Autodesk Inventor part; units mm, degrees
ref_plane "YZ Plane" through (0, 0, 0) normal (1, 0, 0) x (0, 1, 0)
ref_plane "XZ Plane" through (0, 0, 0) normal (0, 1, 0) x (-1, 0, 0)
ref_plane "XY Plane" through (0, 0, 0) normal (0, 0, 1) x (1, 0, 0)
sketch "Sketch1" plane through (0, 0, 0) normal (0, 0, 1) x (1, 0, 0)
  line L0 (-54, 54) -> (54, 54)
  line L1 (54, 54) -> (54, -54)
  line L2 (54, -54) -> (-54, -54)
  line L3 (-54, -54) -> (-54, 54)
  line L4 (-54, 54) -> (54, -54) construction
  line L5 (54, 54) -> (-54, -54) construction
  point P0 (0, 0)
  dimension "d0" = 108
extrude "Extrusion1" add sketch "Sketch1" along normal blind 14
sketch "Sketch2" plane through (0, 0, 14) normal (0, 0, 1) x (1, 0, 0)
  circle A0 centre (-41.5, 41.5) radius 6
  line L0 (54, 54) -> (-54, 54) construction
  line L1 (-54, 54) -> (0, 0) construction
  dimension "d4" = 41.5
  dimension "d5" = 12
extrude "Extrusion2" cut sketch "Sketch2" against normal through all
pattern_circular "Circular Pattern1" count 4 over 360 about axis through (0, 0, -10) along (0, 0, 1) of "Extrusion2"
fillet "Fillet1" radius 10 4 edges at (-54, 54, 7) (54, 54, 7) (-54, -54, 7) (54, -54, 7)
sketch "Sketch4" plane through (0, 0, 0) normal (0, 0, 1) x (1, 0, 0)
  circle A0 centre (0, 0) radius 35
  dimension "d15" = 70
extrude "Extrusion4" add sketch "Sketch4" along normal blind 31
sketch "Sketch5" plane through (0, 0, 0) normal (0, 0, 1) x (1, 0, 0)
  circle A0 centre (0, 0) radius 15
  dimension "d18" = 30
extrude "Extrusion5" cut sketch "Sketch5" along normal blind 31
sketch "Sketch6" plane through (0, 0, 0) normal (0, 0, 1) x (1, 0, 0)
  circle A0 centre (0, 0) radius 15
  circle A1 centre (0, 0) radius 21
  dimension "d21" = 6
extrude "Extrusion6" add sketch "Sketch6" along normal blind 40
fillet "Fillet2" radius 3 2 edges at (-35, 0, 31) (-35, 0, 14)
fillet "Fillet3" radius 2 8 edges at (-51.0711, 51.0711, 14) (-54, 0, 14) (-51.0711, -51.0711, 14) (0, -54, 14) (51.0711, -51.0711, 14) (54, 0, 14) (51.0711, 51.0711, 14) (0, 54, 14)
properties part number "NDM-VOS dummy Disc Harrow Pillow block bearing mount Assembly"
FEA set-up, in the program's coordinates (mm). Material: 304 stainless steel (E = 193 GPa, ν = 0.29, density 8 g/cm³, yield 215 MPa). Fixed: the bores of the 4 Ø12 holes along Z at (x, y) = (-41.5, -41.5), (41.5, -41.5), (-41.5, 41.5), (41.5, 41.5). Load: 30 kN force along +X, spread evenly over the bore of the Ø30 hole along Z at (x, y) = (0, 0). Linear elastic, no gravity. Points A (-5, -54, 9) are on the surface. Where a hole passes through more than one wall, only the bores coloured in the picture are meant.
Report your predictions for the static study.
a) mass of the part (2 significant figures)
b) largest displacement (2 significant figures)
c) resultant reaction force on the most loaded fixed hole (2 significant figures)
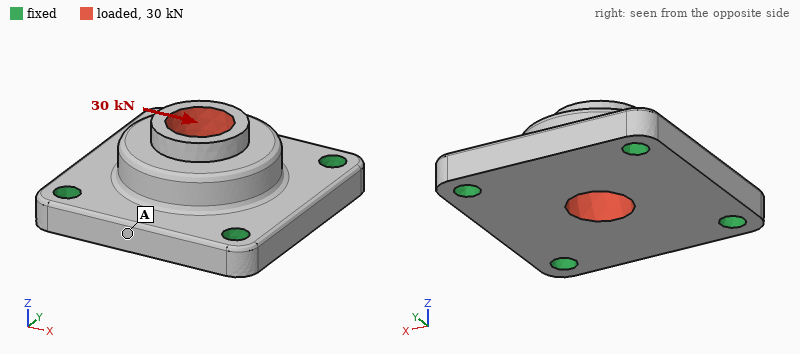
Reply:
1.6 kg
12 µm
8.6 kN
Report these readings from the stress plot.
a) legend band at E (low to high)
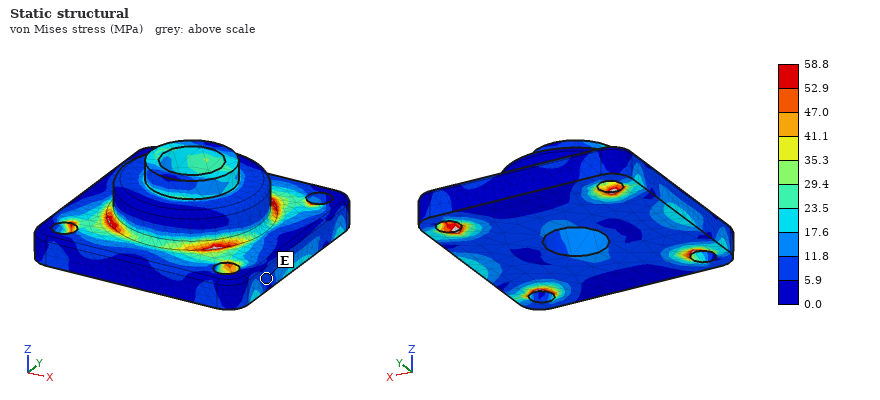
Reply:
5.9 to 11.8 MPa
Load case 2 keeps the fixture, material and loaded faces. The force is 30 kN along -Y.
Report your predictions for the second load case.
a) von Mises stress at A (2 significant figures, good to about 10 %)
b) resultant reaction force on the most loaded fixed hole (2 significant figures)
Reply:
11 MPa
8.6 kN
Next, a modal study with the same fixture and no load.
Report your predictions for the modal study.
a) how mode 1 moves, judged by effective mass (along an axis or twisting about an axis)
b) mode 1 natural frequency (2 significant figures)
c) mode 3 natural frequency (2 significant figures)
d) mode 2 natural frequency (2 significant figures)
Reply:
along Z
7000 Hz
9400 Hz
9400 Hz
